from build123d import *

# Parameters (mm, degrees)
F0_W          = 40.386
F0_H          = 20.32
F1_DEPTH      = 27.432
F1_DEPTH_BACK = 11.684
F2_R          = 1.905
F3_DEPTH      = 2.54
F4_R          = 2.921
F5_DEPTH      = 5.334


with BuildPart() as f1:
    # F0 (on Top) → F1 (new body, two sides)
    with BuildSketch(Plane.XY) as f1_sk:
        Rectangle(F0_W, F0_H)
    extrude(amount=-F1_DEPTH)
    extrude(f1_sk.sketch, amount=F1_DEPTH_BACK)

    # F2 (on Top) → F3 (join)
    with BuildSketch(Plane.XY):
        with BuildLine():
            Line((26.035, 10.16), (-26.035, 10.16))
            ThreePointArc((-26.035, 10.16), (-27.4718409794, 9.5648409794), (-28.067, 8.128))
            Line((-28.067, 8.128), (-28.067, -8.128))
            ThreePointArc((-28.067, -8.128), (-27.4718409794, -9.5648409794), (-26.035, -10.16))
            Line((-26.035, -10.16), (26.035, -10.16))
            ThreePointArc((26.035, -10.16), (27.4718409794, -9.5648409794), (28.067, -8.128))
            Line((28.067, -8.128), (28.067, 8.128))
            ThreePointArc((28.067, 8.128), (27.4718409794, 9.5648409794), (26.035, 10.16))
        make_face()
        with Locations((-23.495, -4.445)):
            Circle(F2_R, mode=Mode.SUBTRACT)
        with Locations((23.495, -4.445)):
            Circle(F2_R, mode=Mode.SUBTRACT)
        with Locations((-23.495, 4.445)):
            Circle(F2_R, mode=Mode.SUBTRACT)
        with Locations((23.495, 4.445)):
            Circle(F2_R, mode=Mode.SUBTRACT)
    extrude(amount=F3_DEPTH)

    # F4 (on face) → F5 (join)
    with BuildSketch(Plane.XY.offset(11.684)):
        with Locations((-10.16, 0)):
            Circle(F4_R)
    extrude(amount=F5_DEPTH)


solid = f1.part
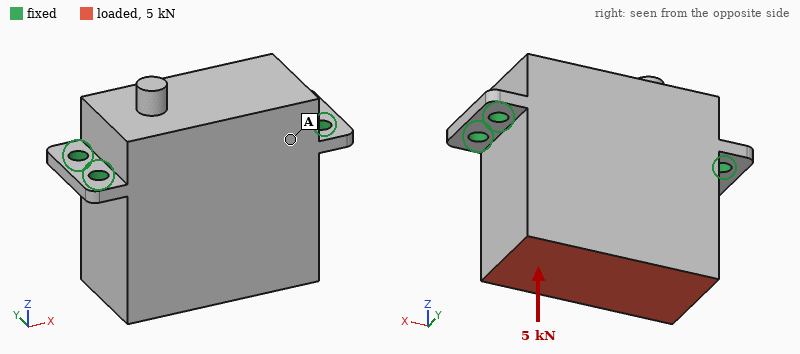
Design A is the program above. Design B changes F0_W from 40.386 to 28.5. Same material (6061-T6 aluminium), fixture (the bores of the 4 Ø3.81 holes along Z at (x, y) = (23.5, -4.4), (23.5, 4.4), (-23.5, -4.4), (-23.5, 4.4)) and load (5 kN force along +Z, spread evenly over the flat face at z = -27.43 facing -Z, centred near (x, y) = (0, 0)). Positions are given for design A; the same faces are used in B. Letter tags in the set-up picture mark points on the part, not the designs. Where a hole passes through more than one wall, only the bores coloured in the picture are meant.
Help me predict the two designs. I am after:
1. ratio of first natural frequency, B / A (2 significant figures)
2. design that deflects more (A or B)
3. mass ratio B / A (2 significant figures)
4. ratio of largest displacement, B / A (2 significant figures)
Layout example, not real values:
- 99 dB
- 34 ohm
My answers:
- 0.50
- B
- 0.73
- 6.8
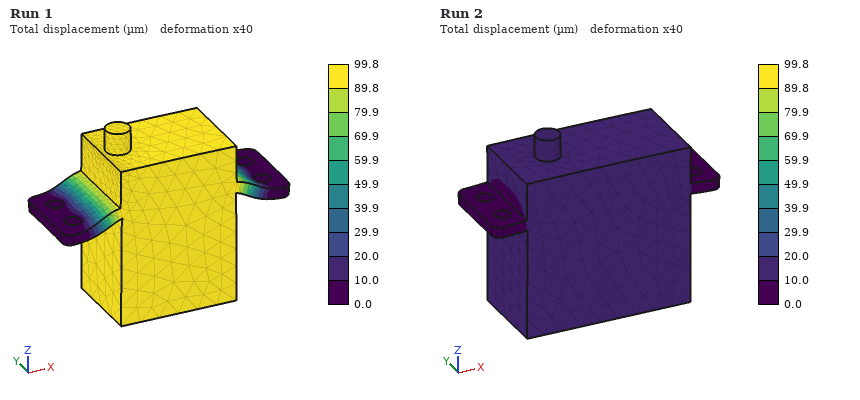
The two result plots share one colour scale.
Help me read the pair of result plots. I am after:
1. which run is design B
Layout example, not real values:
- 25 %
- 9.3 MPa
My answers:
- Run 1
